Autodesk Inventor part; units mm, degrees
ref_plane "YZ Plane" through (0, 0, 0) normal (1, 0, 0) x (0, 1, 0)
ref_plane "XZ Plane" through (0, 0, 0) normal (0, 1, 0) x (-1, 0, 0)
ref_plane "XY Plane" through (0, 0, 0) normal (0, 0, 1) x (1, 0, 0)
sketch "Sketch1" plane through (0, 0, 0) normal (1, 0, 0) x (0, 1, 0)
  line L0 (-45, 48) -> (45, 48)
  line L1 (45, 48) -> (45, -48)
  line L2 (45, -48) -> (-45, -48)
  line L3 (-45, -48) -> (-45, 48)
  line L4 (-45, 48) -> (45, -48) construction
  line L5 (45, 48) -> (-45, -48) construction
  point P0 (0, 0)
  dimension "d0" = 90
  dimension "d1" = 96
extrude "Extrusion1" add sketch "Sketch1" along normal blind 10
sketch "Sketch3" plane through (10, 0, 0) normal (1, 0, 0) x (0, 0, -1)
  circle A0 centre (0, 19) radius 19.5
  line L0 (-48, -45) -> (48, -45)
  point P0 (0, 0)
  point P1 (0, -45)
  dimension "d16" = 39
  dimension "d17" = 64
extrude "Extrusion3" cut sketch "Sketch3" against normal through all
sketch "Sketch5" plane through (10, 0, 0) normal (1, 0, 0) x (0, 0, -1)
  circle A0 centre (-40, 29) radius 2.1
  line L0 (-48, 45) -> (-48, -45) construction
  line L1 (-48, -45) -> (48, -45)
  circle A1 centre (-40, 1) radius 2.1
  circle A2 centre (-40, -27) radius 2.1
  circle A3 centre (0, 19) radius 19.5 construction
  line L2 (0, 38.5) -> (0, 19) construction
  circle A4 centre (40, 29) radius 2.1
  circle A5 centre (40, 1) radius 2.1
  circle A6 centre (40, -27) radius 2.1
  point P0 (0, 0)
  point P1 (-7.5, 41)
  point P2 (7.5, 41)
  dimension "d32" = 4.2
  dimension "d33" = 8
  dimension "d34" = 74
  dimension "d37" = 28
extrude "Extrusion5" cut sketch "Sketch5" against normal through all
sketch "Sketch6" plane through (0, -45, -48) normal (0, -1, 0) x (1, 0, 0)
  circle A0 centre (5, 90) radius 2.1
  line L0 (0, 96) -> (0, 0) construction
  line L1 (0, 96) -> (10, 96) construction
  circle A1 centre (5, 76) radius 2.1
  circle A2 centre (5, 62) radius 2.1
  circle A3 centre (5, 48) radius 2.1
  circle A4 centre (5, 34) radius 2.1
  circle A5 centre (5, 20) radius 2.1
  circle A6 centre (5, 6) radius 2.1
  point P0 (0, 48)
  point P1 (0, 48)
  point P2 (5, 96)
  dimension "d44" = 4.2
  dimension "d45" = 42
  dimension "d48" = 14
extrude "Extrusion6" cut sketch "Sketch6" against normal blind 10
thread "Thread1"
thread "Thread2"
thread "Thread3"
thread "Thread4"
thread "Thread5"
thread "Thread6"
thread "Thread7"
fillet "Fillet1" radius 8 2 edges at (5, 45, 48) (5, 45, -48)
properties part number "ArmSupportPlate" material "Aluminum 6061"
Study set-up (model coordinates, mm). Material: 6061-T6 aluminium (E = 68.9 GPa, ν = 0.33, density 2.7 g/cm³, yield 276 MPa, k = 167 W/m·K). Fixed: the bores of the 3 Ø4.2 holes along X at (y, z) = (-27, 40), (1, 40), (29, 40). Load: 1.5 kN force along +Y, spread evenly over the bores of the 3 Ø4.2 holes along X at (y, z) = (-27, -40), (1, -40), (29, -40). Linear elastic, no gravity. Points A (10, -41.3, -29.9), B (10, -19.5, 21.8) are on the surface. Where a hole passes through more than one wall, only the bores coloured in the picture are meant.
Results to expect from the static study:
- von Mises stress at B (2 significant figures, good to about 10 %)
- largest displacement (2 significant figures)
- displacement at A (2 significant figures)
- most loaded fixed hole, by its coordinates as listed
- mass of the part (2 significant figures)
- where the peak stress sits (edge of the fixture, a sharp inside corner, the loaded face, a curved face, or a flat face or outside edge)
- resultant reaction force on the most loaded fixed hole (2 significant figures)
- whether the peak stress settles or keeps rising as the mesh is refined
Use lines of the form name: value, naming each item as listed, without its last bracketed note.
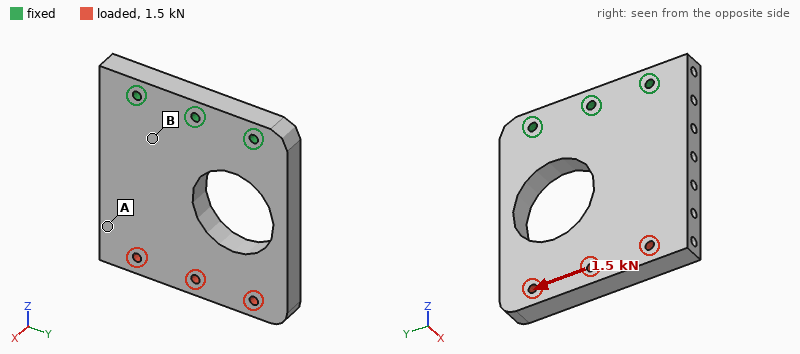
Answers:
von Mises stress at B: 7.4 MPa
largest displacement: 36 µm
displacement at A: 28 µm
most loaded fixed hole, by its coordinates as listed: (-27, 40)
mass of the part: 200 g
where the peak stress sits: edge of the fixture
resultant reaction force on the most loaded fixed hole: 2.4 kN
whether the peak stress settles or keeps rising as the mesh is refined: keeps rising
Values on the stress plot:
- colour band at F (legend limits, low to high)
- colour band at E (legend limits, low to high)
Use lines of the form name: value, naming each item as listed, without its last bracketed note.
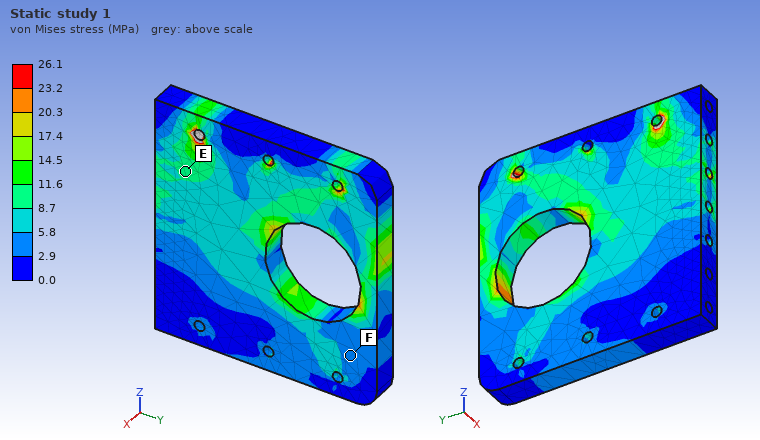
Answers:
colour band at F: 2.9 to 5.8 MPa
colour band at E: 8.7 to 11.6 MPa
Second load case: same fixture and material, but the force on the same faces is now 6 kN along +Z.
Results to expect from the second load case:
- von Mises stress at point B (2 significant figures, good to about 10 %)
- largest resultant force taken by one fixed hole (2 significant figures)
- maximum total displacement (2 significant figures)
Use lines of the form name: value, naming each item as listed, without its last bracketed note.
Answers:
von Mises stress at point B: 11 MPa
largest resultant force taken by one fixed hole: 2.3 kN
maximum total displacement: 28 µm
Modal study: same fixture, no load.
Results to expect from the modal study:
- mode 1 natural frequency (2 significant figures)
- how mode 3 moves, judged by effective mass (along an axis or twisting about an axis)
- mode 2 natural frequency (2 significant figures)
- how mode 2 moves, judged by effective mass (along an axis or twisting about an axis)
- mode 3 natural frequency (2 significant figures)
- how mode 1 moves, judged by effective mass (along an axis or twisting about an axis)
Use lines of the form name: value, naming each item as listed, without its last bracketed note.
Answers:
mode 1 natural frequency: 910 Hz
how mode 3 moves, judged by effective mass: along Y
mode 2 natural frequency: 2100 Hz
how mode 2 moves, judged by effective mass: twisting about Z
mode 3 natural frequency: 4000 Hz
how mode 1 moves, judged by effective mass: along X
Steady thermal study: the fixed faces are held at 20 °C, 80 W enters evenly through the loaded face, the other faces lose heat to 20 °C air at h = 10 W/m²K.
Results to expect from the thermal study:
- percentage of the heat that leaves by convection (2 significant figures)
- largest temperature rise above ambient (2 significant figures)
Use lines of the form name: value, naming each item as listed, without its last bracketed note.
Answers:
percentage of the heat that leaves by convection: 7.9 %
largest temperature rise above ambient: 68 K
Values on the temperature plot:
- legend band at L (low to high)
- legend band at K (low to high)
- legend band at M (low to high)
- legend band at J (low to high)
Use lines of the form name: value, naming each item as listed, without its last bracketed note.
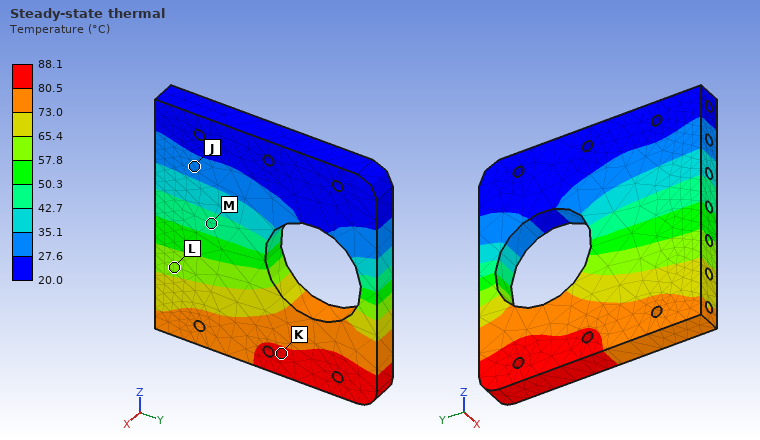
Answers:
legend band at L: 57.8 to 65.4 °C
legend band at K: 80.5 to 88.1 °C
legend band at M: 42.7 to 50.3 °C
legend band at J: 27.6 to 35.1 °C
